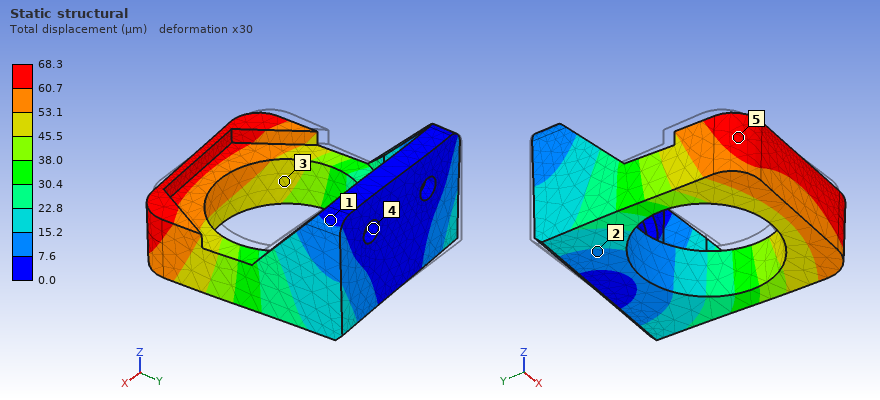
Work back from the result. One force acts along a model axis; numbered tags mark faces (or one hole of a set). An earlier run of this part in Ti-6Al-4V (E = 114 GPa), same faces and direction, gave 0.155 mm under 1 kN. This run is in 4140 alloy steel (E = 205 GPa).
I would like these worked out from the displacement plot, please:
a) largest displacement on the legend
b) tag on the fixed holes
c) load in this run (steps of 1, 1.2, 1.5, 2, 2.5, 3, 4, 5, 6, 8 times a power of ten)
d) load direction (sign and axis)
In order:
68.3 µm
4
800 N
+X
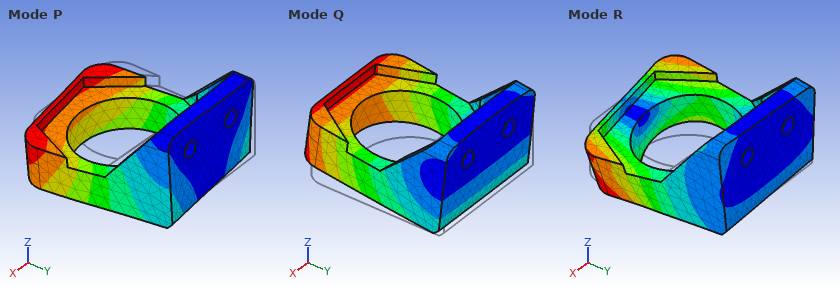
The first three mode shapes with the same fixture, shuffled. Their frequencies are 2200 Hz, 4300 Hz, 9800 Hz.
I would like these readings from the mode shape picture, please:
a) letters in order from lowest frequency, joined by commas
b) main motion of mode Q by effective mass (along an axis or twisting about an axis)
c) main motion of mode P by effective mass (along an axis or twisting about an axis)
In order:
Q, P, R
along Z
along X
